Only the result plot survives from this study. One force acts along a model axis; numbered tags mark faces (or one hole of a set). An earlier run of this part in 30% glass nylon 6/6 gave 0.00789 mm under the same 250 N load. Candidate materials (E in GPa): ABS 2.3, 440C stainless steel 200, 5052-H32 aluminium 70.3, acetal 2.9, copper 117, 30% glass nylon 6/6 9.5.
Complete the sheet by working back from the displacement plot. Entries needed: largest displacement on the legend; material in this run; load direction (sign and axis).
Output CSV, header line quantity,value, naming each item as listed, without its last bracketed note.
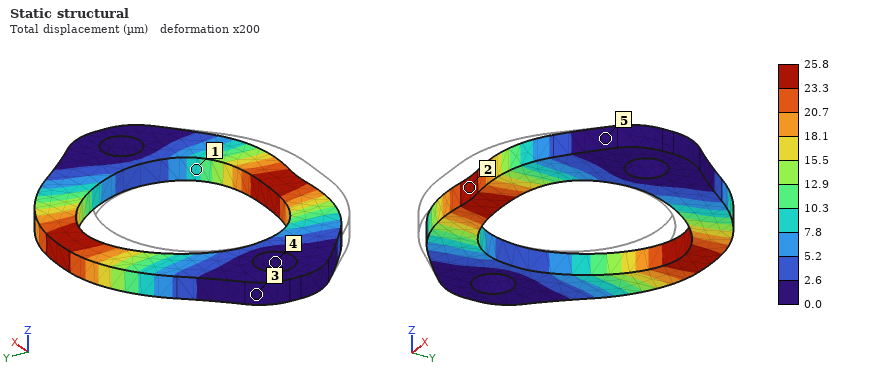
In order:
quantity,value
largest displacement on the legend,25.8 µm
material in this run,acetal
load direction,+Y
